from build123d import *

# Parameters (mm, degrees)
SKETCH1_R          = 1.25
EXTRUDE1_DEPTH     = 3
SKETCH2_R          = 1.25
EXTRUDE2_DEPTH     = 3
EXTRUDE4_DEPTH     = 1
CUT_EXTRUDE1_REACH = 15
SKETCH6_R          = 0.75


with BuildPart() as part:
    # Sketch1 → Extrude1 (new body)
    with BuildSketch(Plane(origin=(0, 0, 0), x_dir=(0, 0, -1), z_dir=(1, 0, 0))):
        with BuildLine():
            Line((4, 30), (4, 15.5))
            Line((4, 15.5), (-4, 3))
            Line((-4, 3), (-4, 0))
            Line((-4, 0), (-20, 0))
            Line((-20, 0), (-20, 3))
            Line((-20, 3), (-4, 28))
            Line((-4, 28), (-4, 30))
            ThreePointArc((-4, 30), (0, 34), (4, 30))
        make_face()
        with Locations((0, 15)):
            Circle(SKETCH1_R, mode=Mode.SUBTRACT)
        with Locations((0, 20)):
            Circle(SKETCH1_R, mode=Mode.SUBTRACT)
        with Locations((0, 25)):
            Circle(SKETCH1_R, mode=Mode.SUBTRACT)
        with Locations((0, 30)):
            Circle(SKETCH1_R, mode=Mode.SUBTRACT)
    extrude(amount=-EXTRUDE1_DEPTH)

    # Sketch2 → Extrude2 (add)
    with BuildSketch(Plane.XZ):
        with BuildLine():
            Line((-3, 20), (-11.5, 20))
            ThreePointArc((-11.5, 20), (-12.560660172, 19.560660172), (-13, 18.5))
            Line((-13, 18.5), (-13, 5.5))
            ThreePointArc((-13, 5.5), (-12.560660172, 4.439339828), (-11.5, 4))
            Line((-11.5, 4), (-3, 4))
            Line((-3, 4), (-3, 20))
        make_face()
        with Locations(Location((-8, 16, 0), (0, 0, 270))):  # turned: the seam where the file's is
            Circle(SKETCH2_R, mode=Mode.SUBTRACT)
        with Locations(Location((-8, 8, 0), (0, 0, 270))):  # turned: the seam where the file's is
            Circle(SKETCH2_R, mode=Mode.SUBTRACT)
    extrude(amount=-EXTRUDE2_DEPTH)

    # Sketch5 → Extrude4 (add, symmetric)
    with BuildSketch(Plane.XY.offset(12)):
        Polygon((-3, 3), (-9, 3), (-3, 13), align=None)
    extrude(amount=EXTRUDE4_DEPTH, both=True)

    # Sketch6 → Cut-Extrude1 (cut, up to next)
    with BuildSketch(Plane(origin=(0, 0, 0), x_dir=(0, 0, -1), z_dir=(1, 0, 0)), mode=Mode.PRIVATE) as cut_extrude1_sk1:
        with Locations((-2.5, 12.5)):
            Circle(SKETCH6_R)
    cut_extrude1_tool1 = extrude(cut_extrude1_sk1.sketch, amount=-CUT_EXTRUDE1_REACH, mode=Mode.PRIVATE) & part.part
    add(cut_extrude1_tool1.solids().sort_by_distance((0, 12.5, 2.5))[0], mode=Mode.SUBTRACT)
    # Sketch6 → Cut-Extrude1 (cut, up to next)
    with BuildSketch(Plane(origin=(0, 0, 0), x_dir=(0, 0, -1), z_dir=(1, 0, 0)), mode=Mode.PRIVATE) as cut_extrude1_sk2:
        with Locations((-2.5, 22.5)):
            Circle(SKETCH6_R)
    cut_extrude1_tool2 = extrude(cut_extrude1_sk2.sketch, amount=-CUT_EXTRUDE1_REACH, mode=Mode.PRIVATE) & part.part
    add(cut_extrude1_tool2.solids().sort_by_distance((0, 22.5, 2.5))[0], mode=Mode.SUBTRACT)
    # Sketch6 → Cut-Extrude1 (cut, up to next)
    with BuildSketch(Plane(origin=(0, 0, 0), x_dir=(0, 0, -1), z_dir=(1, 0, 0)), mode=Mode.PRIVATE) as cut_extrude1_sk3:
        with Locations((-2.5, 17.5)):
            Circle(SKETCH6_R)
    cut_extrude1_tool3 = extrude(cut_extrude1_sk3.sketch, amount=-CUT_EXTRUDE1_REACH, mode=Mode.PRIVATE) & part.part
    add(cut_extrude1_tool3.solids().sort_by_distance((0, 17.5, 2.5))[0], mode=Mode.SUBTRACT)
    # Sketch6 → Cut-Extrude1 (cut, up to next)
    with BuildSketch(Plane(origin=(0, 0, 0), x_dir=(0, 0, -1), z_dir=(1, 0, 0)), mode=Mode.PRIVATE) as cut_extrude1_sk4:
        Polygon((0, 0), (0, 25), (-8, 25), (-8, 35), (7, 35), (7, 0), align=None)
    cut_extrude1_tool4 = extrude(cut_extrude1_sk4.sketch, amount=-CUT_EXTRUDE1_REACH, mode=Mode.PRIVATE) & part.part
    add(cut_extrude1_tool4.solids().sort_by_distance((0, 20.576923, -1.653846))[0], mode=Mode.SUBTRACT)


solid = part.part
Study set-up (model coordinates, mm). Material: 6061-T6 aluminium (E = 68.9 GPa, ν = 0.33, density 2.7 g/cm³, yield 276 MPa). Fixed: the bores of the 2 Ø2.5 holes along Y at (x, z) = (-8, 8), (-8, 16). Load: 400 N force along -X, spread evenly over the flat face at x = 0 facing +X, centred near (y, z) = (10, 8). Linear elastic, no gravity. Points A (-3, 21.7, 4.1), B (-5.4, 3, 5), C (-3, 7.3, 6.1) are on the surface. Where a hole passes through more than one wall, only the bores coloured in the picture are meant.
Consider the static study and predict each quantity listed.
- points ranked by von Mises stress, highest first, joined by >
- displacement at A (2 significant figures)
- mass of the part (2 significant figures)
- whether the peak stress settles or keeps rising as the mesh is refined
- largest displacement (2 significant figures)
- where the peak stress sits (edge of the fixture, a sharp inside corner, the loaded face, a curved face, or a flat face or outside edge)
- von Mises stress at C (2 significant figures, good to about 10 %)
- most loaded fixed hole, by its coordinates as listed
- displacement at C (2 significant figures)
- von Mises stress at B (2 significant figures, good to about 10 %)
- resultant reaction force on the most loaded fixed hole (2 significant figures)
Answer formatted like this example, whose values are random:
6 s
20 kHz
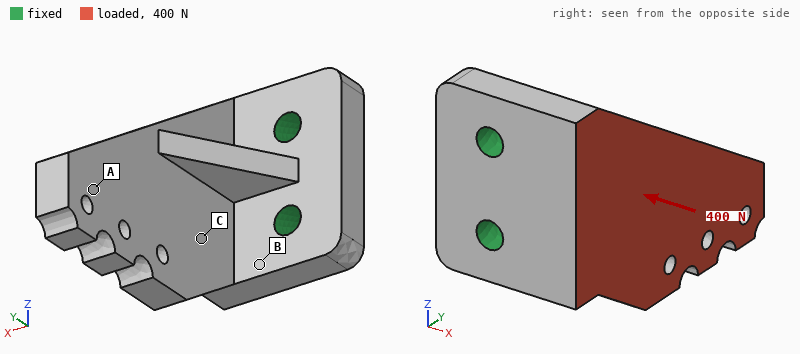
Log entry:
B > C > A
0.18 mm
3.9 g
keeps rising
0.23 mm
edge of the fixture
55 MPa
(-8, 8)
0.039 mm
100 MPa
350 N
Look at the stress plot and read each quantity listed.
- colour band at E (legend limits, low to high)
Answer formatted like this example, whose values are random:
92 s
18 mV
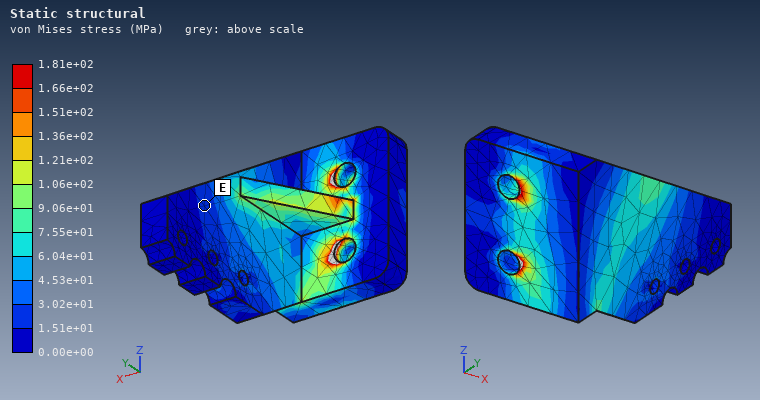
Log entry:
1.51e+01 to 3.02e+01 MPa
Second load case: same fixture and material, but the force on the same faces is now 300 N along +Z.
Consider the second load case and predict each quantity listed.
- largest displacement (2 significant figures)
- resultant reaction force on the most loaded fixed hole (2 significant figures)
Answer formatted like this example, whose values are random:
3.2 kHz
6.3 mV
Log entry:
49 µm
390 N
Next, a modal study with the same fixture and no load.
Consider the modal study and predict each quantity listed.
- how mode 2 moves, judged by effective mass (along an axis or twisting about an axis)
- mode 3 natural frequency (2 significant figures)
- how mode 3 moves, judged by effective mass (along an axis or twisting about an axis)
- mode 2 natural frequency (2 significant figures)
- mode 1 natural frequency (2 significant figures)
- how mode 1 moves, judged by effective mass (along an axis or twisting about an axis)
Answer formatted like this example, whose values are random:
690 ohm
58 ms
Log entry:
along Z
18 kHz
along Y
9500 Hz
5500 Hz
along X
